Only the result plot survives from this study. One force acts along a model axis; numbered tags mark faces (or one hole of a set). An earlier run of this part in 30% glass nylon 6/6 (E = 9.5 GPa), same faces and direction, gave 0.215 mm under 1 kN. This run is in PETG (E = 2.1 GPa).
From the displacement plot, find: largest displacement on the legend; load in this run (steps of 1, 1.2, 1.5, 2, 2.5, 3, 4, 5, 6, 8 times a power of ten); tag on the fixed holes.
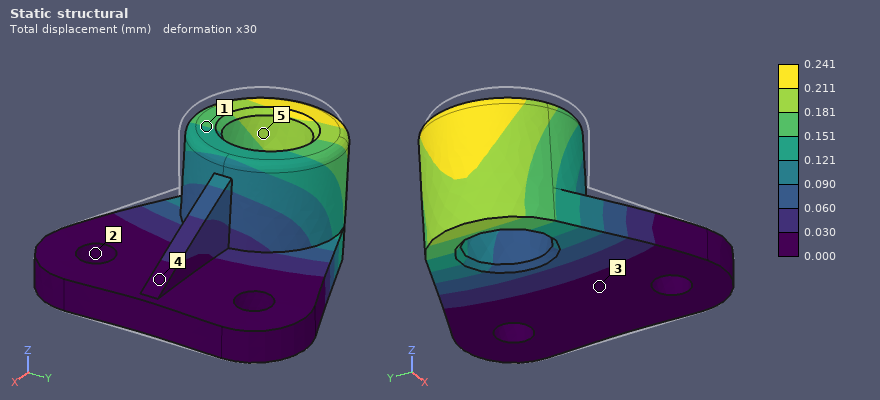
0.241 mm
250 N
2
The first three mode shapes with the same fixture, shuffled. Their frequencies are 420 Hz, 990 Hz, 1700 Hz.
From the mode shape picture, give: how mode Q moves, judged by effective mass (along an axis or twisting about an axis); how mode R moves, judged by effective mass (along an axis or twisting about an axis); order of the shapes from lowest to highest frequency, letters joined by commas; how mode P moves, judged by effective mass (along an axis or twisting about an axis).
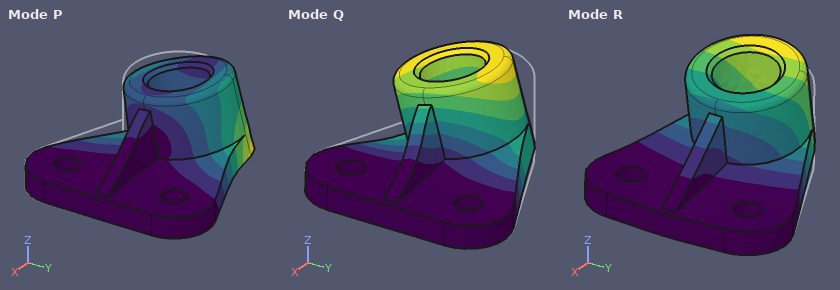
along Y
along Z
R, Q, P
along Y
